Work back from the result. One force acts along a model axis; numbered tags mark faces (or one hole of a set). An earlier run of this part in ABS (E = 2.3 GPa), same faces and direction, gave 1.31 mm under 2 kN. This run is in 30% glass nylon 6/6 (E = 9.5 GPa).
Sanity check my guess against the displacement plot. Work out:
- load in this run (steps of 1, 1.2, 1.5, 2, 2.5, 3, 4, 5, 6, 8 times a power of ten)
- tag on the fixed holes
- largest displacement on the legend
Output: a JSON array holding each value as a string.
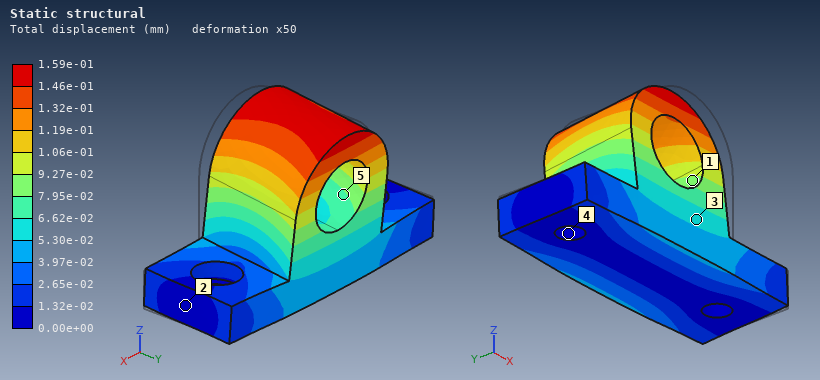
["1 kN", "4", "1.59e-01 mm"]
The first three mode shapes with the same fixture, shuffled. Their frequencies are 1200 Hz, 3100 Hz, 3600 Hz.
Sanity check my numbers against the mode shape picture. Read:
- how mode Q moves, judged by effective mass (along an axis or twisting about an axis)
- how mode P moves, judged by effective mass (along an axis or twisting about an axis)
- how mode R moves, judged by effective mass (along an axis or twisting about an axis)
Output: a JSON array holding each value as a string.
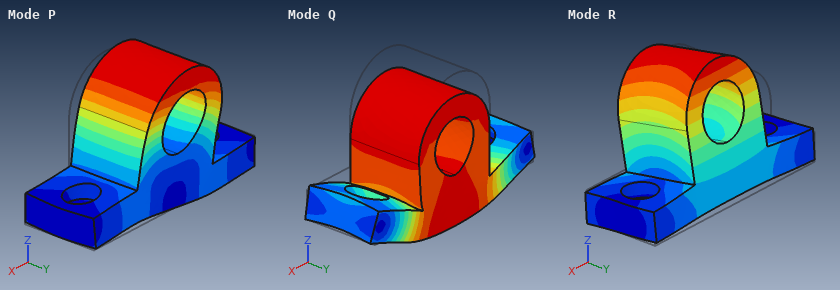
["along Z", "along X", "along Y"]
